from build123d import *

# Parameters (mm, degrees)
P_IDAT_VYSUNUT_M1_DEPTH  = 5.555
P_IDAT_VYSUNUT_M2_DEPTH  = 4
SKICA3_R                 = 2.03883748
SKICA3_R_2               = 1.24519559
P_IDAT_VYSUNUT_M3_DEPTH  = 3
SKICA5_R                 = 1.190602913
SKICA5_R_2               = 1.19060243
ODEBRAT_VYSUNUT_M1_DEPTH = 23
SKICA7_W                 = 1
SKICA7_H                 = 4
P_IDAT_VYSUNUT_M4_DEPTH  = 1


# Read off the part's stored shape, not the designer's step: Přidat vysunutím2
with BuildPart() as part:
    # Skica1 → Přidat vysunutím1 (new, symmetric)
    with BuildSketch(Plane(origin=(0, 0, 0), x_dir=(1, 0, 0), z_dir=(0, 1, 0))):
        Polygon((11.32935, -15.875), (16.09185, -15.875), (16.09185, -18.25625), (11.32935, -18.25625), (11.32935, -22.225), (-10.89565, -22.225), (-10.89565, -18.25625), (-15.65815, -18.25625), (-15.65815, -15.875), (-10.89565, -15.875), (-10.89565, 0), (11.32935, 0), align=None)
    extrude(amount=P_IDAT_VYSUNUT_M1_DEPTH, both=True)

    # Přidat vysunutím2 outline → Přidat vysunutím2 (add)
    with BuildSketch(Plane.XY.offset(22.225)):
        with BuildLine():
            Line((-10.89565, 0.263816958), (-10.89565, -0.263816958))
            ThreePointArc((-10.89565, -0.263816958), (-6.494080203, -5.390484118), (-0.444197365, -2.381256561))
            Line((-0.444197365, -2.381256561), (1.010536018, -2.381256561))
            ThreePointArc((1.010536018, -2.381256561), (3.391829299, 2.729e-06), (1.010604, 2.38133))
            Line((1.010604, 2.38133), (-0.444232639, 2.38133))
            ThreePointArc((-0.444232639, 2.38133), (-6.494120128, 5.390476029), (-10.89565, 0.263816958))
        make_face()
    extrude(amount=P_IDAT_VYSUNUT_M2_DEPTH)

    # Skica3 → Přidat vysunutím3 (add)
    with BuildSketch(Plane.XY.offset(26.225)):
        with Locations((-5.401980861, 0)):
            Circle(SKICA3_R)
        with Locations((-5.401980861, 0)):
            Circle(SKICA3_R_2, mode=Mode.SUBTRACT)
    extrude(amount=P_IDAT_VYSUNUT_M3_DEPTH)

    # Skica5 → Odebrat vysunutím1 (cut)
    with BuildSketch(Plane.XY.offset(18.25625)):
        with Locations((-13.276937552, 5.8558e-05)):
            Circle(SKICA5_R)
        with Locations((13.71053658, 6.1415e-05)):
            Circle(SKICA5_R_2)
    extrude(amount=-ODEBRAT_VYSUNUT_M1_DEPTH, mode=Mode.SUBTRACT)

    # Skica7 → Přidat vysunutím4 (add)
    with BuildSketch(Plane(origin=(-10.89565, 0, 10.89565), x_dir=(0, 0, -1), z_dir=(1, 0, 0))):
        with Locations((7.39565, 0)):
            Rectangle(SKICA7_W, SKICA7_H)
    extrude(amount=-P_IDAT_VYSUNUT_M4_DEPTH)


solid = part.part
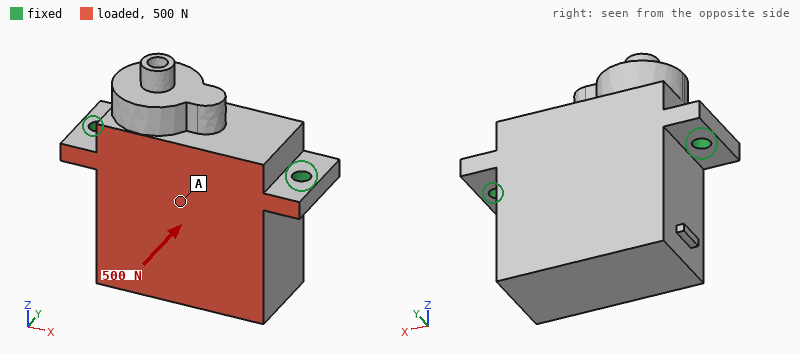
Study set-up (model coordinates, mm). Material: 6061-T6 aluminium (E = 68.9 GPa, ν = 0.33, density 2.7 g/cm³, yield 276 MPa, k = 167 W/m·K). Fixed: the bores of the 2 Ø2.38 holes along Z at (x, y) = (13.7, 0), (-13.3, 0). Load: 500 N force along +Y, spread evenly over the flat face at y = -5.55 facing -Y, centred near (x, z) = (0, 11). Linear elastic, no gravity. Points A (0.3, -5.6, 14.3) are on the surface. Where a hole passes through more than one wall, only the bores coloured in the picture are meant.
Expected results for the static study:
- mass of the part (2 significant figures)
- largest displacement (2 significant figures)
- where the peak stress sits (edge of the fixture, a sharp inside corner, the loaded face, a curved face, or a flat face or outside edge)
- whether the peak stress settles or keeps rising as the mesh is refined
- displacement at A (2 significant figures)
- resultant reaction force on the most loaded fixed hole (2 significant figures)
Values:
17 g
54 µm
edge of the fixture
keeps rising
19 µm
250 N
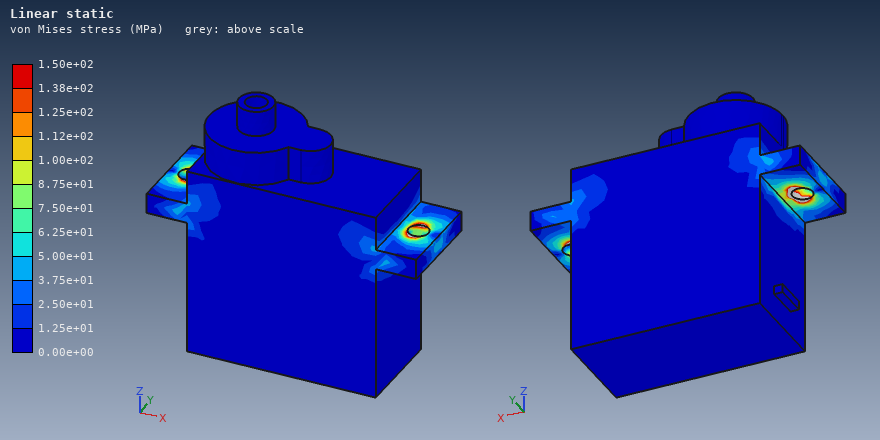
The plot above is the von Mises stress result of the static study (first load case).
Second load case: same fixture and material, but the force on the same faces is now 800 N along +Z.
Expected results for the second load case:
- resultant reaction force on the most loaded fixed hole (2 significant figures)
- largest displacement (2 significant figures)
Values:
400 N
79 µm
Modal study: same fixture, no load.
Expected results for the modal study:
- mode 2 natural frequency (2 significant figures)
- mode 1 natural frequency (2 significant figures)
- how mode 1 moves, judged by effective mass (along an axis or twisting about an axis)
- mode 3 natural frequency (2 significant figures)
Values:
17 kHz
4300 Hz
along Y
18 kHz
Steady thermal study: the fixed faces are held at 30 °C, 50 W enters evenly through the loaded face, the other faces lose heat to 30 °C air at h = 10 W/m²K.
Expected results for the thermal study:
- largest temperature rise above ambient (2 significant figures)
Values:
33 K
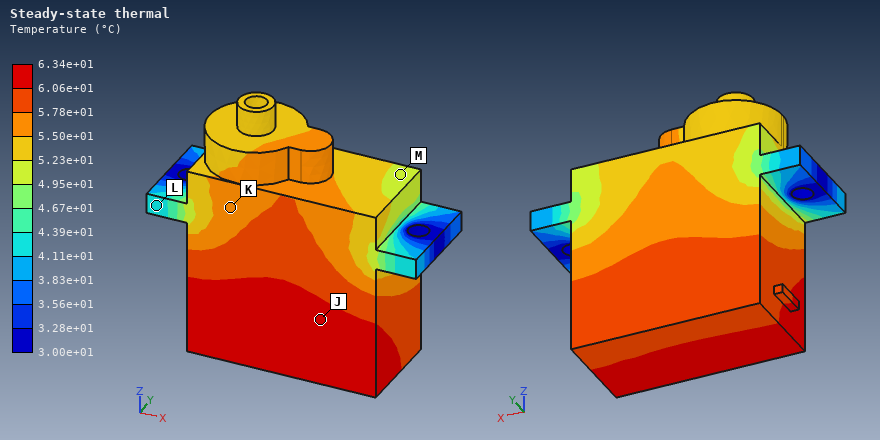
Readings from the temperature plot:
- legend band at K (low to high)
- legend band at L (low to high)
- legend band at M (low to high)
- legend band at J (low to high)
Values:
5.50e+01 to 5.78e+01 °C
4.11e+01 to 4.39e+01 °C
4.95e+01 to 5.23e+01 °C
6.06e+01 to 6.34e+01 °C
